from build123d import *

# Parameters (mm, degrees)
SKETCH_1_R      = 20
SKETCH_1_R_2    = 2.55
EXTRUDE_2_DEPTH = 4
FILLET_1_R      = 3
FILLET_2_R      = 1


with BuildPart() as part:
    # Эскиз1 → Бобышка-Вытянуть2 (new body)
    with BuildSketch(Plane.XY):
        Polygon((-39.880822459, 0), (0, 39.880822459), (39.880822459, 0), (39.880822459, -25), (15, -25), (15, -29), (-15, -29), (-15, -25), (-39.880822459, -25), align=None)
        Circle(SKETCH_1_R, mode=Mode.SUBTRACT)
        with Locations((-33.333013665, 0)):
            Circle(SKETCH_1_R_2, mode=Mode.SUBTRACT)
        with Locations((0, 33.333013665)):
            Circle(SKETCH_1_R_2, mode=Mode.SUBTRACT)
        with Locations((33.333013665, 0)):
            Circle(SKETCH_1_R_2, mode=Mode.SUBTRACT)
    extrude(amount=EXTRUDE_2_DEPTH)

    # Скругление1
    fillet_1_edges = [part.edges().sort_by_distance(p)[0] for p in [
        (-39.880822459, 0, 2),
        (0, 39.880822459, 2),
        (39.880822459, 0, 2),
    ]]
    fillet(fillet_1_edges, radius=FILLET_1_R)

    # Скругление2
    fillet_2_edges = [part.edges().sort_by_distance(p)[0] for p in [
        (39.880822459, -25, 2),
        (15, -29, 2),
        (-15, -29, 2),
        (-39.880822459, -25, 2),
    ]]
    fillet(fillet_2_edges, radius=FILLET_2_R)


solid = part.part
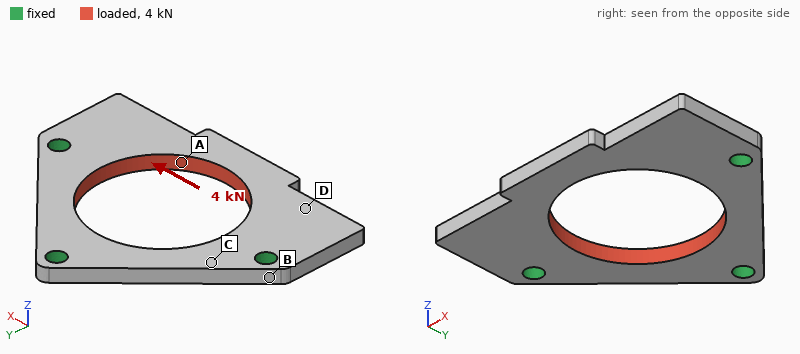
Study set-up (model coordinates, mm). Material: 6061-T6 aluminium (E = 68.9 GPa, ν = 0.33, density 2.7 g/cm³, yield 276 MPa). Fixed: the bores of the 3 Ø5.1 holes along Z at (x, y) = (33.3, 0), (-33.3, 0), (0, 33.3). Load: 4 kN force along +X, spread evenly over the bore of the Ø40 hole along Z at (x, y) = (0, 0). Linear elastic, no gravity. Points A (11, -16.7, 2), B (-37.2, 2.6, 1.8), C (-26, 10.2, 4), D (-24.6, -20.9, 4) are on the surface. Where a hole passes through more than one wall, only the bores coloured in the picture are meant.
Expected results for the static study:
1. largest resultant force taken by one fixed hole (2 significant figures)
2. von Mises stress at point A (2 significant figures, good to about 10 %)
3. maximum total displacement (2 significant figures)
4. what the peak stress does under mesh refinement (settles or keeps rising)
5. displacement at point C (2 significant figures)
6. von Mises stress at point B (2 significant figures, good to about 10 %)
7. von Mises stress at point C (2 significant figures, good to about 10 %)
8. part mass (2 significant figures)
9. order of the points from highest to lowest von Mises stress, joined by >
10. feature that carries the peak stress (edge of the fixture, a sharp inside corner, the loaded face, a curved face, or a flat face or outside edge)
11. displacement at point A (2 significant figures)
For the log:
1.6 kN
43 MPa
20 µm
keeps rising
4.6 µm
33 MPa
16 MPa
26 g
A > B > C > D
edge of the fixture
19 µm
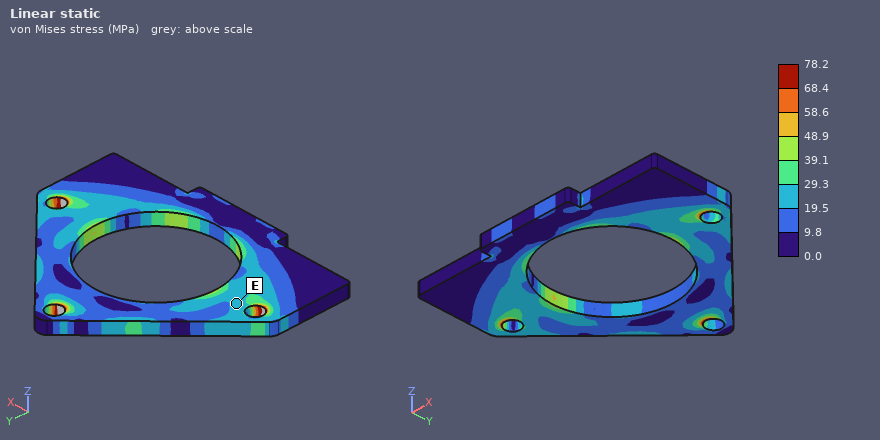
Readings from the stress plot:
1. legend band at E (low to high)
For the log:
19.5 to 29.3 MPa
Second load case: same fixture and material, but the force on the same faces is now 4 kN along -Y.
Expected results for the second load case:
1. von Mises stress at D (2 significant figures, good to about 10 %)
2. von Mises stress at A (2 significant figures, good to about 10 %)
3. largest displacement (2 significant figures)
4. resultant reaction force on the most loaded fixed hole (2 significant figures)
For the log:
11 MPa
21 MPa
21 µm
1.6 kN
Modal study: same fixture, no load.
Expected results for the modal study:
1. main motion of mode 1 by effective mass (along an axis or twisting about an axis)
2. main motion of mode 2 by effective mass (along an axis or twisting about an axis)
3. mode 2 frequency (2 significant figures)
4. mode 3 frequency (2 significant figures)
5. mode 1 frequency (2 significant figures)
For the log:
along Z
twisting about Y
5600 Hz
7900 Hz
2900 Hz
